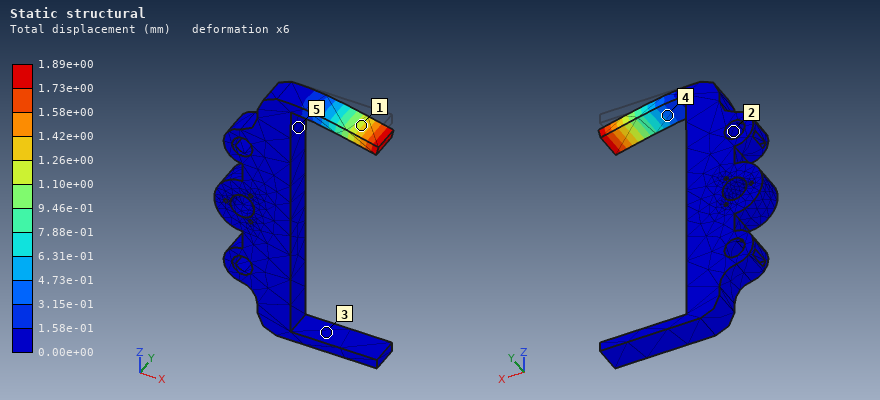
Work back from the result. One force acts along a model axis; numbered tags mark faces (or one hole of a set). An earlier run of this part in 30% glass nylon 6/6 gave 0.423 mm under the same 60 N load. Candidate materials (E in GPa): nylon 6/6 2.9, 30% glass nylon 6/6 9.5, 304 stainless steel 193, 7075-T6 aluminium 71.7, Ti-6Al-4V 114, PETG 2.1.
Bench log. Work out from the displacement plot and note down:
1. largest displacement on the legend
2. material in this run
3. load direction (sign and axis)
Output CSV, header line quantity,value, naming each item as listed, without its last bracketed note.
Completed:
quantity,value
largest displacement on the legend,1.89e+00 mm
material in this run,PETG
load direction,-Z
